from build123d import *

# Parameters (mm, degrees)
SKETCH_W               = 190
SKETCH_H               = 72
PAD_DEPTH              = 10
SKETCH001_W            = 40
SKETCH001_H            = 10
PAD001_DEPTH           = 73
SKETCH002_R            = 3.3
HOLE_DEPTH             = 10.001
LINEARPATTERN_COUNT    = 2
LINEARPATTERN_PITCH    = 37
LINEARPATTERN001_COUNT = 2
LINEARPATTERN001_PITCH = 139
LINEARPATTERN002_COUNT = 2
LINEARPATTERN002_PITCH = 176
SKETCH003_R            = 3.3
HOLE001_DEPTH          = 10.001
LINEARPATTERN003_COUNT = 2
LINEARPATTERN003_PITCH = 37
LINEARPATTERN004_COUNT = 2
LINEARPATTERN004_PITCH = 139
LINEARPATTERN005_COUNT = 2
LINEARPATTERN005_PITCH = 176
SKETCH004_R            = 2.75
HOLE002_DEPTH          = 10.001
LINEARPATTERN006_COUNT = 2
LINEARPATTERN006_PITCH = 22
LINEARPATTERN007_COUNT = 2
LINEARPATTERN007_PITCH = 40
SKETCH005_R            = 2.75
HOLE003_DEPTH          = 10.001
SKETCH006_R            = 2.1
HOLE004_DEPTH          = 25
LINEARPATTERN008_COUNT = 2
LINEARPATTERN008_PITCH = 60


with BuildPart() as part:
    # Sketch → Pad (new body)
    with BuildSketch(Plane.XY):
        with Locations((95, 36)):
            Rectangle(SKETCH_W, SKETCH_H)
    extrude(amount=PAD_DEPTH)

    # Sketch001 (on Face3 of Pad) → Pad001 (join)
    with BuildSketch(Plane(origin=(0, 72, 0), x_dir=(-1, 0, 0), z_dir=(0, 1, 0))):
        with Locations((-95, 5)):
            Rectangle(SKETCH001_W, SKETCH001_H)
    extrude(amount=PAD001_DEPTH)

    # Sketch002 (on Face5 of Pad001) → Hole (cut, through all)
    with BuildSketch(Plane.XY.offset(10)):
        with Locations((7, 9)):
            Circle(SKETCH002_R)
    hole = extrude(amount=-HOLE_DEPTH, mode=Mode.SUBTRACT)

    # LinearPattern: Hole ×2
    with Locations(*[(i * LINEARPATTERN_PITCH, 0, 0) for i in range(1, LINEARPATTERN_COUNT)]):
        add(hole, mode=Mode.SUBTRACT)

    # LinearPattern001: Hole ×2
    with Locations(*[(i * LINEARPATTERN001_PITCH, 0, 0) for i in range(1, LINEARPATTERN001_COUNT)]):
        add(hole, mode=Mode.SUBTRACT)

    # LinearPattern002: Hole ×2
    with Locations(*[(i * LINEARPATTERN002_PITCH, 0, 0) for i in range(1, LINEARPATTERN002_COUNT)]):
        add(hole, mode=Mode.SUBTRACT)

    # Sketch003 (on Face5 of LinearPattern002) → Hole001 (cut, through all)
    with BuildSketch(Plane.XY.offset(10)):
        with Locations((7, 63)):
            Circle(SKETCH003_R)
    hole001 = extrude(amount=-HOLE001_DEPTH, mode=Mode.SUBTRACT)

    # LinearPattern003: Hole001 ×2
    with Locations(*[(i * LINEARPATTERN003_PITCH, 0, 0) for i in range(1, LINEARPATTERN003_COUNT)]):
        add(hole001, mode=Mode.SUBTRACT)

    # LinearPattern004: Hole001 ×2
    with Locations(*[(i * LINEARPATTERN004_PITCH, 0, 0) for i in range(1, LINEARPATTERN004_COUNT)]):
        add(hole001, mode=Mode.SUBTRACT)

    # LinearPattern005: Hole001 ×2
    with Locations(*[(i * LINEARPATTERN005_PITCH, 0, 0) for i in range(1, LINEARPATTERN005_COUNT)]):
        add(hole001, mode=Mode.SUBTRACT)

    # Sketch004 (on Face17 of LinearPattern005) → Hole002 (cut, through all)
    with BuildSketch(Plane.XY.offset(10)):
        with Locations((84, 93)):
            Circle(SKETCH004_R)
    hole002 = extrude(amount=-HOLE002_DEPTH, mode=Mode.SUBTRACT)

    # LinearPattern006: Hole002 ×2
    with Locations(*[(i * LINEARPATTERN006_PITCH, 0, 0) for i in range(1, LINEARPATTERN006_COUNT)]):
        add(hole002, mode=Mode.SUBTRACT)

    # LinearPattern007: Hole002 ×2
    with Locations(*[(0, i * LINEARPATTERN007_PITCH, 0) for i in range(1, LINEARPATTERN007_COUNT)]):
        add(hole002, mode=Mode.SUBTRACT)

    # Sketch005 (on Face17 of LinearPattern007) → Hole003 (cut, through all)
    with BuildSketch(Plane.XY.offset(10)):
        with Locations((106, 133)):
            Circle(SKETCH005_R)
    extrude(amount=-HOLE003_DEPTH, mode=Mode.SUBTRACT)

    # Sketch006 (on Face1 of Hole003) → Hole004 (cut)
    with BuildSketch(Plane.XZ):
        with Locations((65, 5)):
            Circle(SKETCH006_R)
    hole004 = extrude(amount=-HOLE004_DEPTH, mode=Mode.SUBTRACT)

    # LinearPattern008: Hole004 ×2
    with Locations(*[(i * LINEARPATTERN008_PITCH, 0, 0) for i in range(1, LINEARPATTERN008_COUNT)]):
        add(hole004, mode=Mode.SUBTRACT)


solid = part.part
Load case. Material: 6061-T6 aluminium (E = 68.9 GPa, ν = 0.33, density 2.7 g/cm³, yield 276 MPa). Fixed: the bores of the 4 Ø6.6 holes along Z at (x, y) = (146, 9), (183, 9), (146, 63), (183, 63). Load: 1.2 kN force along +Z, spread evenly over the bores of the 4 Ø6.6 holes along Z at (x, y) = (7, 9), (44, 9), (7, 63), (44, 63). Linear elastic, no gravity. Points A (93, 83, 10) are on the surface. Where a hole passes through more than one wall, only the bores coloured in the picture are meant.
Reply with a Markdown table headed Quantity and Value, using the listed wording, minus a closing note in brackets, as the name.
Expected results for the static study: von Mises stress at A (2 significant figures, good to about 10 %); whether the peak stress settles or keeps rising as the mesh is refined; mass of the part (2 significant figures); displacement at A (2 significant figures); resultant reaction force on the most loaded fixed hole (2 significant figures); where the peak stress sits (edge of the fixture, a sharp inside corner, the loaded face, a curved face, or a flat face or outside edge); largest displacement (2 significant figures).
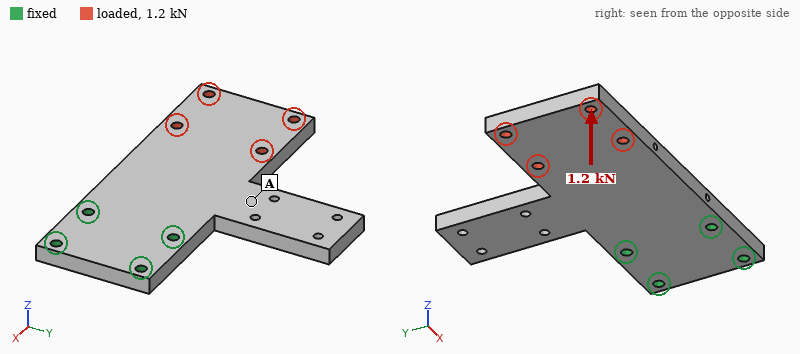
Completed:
| Quantity | Value |
|---|---|
| von Mises stress at A | 22 MPa |
| whether the peak stress settles or keeps rising as the mesh is refined | keeps rising |
| mass of the part | 440 g |
| displacement at A | 0.43 mm |
| resultant reaction force on the most loaded fixed hole | 1.3 kN |
| where the peak stress sits | edge of the fixture |
| largest displacement | 2.3 mm |
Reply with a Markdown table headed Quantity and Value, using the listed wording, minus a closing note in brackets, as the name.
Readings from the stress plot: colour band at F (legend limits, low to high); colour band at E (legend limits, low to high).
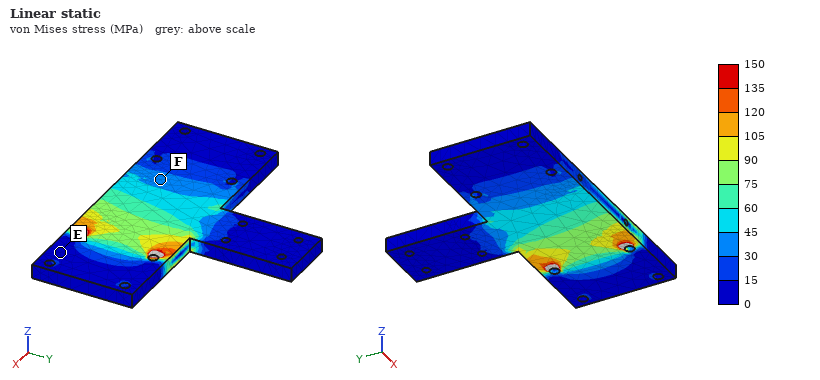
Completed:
| Quantity | Value |
|---|---|
| colour band at F | 30 to 45 MPa |
| colour band at E | 0 to 15 MPa |
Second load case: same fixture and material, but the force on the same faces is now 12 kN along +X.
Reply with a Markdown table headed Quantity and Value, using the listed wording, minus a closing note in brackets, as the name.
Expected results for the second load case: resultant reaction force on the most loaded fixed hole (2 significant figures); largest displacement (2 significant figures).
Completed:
| Quantity | Value |
|---|---|
| resultant reaction force on the most loaded fixed hole | 5.1 kN |
| largest displacement | 41 µm |
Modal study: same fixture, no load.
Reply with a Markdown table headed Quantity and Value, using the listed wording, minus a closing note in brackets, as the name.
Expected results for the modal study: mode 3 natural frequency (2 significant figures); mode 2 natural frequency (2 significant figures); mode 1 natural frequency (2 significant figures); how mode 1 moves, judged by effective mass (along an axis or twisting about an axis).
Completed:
| Quantity | Value |
|---|---|
| mode 3 natural frequency | 1900 Hz |
| mode 2 natural frequency | 740 Hz |
| mode 1 natural frequency | 380 Hz |
| how mode 1 moves, judged by effective mass | along Z |
